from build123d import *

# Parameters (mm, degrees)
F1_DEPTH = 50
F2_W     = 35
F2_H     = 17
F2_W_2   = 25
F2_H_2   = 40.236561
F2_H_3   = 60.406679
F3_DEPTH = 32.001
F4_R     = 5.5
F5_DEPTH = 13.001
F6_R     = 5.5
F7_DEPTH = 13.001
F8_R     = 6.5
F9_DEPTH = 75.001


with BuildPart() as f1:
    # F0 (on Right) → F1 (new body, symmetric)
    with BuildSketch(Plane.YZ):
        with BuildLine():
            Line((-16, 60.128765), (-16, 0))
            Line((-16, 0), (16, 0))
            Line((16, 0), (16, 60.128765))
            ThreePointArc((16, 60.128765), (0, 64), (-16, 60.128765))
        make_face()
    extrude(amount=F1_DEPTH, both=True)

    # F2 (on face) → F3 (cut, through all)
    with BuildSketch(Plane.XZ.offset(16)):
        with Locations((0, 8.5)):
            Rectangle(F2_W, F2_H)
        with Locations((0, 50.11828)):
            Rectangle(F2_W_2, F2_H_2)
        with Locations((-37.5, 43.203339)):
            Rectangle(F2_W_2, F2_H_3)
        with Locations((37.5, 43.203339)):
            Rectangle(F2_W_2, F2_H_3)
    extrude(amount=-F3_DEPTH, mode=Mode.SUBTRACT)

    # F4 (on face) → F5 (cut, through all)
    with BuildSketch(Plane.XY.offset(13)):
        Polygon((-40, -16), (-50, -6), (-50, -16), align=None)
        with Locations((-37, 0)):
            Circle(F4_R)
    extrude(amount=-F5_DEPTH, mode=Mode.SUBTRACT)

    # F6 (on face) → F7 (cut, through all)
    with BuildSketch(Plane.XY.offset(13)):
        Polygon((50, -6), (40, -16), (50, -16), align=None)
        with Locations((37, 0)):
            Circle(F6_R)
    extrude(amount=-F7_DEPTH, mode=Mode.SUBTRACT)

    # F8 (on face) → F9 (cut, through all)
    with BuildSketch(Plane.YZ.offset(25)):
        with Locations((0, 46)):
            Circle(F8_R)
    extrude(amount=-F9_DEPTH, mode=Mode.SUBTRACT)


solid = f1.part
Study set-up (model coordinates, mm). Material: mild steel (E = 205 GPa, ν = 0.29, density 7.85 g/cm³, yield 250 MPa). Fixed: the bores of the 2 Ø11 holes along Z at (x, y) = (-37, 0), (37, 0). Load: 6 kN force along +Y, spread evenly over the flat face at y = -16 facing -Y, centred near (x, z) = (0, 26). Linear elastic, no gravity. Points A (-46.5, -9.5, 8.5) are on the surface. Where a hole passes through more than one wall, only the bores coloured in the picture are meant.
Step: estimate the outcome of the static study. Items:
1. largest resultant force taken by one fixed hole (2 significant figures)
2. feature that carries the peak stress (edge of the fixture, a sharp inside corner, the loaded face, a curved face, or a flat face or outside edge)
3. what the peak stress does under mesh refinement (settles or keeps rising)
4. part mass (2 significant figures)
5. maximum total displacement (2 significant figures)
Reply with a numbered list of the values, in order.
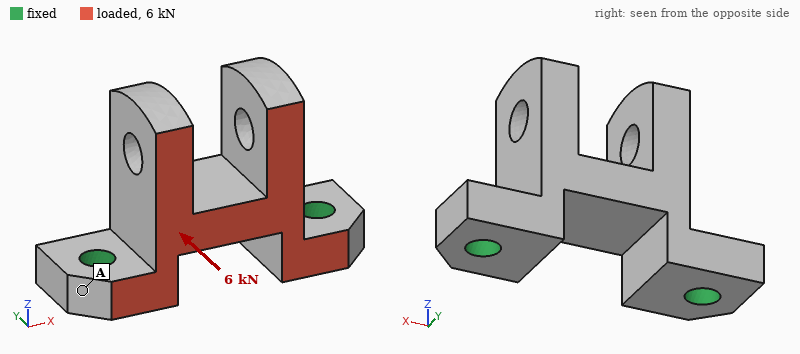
1. 3.0 kN
2. edge of the fixture
3. keeps rising
4. 540 g
5. 39 µm
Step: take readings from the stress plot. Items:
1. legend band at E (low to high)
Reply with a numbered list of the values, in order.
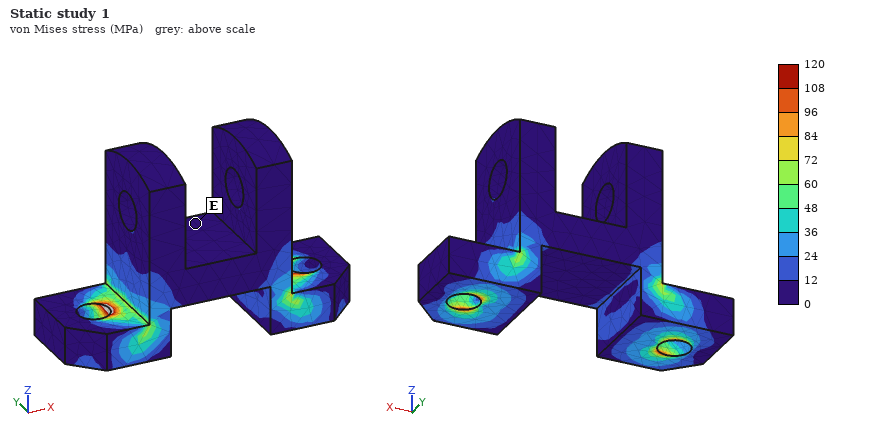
1. 0 to 12 MPa
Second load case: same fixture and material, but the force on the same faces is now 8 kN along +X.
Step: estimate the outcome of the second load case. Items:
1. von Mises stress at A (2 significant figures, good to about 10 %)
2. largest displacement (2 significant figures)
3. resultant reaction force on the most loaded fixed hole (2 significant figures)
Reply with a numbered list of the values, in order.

1. 7.6 MPa
2. 32 µm
3. 4.9 kN
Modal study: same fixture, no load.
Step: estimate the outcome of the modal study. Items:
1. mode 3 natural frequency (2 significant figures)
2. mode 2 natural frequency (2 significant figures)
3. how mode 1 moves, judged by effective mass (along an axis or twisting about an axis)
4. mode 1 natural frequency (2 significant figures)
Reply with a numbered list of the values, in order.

1. 5200 Hz
2. 5100 Hz
3. along Y
4. 3400 Hz
